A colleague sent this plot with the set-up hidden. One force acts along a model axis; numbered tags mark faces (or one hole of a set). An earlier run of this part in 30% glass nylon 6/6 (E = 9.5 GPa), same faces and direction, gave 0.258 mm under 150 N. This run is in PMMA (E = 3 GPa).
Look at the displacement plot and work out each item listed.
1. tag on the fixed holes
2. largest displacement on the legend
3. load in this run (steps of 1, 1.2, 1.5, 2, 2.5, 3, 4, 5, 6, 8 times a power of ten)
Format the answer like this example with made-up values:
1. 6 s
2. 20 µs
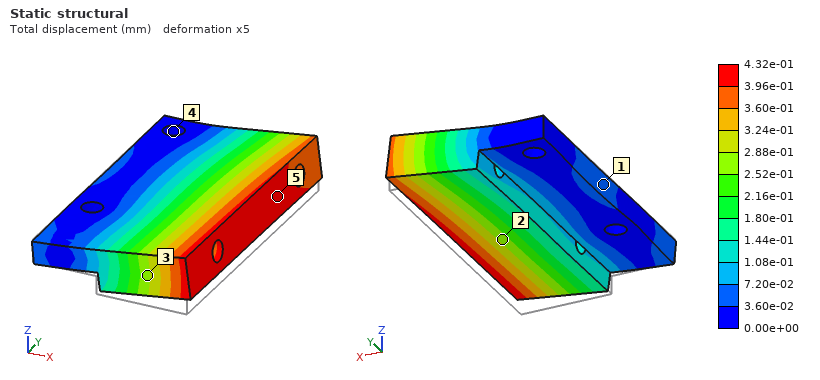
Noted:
1. 4
2. 4.32e-01 mm
3. 80 N
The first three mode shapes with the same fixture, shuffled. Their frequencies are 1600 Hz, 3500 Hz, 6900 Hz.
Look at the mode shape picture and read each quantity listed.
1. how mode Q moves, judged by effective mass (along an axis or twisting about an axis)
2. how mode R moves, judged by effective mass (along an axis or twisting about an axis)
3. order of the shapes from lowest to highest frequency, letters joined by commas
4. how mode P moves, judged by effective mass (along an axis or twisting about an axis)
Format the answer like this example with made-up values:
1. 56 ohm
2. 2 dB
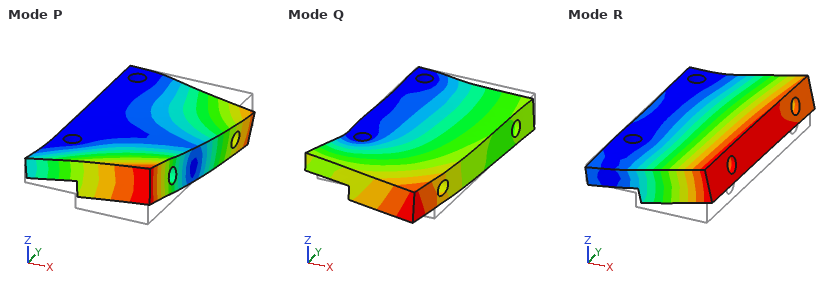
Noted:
1. along Y
2. along Z
3. R, P, Q
4. twisting about X
